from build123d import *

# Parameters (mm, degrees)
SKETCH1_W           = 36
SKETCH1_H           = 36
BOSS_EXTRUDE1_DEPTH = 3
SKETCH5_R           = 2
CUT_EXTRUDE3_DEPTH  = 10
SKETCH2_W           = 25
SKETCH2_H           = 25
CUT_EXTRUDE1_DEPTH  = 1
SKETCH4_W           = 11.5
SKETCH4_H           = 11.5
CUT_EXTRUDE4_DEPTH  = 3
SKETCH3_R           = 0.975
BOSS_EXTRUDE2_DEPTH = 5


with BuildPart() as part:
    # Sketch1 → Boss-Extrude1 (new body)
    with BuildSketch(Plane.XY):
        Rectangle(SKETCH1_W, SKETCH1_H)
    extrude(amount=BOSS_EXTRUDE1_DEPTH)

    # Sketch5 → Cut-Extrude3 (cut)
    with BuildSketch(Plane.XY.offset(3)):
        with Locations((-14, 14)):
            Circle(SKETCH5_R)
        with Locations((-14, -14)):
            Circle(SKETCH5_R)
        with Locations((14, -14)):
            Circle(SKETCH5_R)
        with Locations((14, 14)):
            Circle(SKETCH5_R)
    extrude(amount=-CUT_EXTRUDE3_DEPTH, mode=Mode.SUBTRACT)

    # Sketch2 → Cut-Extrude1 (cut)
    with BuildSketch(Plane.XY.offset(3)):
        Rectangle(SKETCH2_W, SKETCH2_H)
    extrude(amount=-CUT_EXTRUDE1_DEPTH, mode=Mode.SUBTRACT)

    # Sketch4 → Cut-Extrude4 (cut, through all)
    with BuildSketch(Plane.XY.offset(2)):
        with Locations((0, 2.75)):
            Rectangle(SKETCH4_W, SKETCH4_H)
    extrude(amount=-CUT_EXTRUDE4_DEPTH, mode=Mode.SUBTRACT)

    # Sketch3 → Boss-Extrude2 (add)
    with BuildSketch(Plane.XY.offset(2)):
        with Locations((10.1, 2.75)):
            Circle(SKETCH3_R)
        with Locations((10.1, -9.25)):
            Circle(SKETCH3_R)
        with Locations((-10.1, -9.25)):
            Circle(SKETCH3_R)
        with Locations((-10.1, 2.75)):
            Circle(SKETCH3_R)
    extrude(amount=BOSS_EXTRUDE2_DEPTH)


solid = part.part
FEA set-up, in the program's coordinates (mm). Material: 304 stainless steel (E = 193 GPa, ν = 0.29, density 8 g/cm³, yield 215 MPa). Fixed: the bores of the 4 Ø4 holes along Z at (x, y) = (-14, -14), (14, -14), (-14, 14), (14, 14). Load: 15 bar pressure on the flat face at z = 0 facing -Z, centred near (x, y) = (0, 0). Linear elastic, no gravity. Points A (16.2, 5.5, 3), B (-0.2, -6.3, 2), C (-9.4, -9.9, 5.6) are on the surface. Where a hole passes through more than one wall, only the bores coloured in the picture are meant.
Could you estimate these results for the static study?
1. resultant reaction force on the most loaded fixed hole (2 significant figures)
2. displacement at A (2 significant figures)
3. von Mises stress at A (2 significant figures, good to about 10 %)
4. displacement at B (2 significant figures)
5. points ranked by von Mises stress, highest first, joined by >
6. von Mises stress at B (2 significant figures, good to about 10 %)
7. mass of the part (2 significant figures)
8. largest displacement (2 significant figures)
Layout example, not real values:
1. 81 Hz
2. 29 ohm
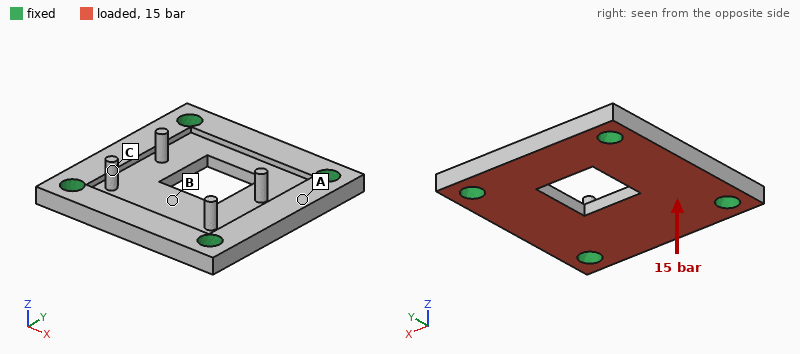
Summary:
1. 440 N
2. 3.9 µm
3. 23 MPa
4. 16 µm
5. B > A > C
6. 38 MPa
7. 23 g
8. 21 µm
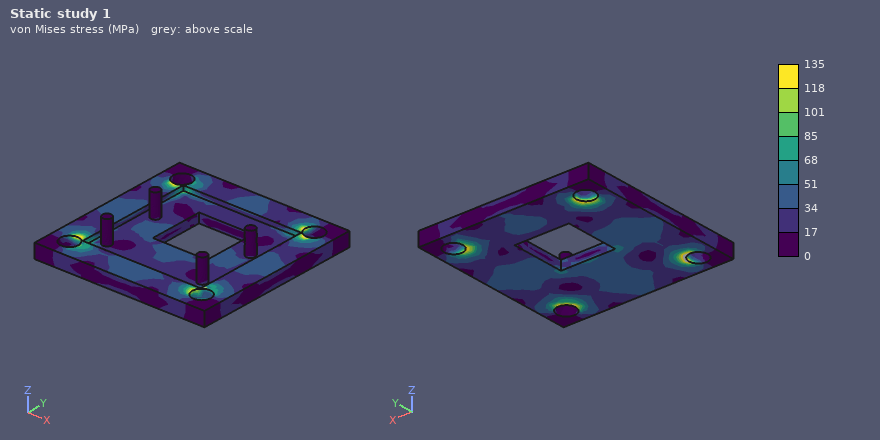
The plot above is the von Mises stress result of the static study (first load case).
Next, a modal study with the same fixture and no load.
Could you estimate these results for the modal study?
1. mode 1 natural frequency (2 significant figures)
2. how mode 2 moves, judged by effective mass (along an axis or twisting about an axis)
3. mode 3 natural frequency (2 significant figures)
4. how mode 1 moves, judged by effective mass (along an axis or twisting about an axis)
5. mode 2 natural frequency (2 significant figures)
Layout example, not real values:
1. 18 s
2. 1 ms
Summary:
1. 14 kHz
2. twisting about Y
3. 21 kHz
4. along Z
5. 20 kHz
